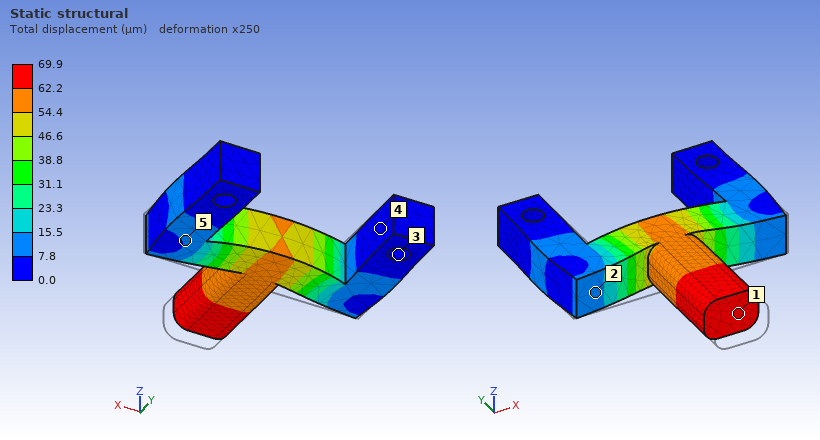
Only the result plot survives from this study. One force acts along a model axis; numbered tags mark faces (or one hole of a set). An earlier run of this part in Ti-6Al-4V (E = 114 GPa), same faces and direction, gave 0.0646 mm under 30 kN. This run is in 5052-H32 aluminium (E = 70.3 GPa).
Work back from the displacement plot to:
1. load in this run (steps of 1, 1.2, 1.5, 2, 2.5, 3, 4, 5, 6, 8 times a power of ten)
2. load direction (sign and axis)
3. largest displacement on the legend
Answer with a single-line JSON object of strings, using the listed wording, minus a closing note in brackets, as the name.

{"load in this run": "20 kN", "load direction": "+Y", "largest displacement on the legend": "69.9 µm"}
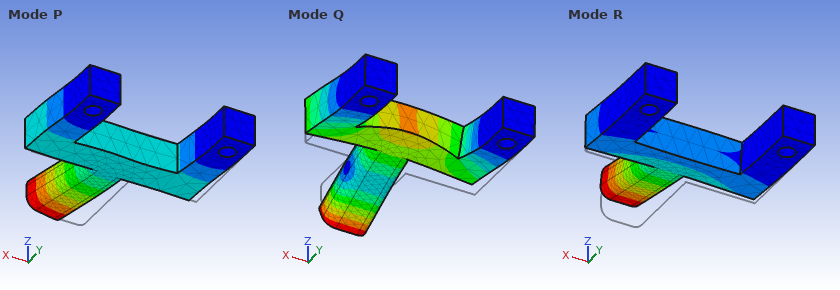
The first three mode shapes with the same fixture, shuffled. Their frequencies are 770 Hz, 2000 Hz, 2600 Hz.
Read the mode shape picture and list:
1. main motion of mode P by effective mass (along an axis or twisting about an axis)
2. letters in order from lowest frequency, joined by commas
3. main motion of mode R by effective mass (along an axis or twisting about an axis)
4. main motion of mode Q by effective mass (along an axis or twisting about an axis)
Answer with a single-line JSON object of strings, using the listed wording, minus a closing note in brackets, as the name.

{"main motion of mode P by effective mass": "along X", "letters in order from lowest frequency, joined by commas": "R, P, Q", "main motion of mode R by effective mass": "along Z", "main motion of mode Q by effective mass": "along Z"}
